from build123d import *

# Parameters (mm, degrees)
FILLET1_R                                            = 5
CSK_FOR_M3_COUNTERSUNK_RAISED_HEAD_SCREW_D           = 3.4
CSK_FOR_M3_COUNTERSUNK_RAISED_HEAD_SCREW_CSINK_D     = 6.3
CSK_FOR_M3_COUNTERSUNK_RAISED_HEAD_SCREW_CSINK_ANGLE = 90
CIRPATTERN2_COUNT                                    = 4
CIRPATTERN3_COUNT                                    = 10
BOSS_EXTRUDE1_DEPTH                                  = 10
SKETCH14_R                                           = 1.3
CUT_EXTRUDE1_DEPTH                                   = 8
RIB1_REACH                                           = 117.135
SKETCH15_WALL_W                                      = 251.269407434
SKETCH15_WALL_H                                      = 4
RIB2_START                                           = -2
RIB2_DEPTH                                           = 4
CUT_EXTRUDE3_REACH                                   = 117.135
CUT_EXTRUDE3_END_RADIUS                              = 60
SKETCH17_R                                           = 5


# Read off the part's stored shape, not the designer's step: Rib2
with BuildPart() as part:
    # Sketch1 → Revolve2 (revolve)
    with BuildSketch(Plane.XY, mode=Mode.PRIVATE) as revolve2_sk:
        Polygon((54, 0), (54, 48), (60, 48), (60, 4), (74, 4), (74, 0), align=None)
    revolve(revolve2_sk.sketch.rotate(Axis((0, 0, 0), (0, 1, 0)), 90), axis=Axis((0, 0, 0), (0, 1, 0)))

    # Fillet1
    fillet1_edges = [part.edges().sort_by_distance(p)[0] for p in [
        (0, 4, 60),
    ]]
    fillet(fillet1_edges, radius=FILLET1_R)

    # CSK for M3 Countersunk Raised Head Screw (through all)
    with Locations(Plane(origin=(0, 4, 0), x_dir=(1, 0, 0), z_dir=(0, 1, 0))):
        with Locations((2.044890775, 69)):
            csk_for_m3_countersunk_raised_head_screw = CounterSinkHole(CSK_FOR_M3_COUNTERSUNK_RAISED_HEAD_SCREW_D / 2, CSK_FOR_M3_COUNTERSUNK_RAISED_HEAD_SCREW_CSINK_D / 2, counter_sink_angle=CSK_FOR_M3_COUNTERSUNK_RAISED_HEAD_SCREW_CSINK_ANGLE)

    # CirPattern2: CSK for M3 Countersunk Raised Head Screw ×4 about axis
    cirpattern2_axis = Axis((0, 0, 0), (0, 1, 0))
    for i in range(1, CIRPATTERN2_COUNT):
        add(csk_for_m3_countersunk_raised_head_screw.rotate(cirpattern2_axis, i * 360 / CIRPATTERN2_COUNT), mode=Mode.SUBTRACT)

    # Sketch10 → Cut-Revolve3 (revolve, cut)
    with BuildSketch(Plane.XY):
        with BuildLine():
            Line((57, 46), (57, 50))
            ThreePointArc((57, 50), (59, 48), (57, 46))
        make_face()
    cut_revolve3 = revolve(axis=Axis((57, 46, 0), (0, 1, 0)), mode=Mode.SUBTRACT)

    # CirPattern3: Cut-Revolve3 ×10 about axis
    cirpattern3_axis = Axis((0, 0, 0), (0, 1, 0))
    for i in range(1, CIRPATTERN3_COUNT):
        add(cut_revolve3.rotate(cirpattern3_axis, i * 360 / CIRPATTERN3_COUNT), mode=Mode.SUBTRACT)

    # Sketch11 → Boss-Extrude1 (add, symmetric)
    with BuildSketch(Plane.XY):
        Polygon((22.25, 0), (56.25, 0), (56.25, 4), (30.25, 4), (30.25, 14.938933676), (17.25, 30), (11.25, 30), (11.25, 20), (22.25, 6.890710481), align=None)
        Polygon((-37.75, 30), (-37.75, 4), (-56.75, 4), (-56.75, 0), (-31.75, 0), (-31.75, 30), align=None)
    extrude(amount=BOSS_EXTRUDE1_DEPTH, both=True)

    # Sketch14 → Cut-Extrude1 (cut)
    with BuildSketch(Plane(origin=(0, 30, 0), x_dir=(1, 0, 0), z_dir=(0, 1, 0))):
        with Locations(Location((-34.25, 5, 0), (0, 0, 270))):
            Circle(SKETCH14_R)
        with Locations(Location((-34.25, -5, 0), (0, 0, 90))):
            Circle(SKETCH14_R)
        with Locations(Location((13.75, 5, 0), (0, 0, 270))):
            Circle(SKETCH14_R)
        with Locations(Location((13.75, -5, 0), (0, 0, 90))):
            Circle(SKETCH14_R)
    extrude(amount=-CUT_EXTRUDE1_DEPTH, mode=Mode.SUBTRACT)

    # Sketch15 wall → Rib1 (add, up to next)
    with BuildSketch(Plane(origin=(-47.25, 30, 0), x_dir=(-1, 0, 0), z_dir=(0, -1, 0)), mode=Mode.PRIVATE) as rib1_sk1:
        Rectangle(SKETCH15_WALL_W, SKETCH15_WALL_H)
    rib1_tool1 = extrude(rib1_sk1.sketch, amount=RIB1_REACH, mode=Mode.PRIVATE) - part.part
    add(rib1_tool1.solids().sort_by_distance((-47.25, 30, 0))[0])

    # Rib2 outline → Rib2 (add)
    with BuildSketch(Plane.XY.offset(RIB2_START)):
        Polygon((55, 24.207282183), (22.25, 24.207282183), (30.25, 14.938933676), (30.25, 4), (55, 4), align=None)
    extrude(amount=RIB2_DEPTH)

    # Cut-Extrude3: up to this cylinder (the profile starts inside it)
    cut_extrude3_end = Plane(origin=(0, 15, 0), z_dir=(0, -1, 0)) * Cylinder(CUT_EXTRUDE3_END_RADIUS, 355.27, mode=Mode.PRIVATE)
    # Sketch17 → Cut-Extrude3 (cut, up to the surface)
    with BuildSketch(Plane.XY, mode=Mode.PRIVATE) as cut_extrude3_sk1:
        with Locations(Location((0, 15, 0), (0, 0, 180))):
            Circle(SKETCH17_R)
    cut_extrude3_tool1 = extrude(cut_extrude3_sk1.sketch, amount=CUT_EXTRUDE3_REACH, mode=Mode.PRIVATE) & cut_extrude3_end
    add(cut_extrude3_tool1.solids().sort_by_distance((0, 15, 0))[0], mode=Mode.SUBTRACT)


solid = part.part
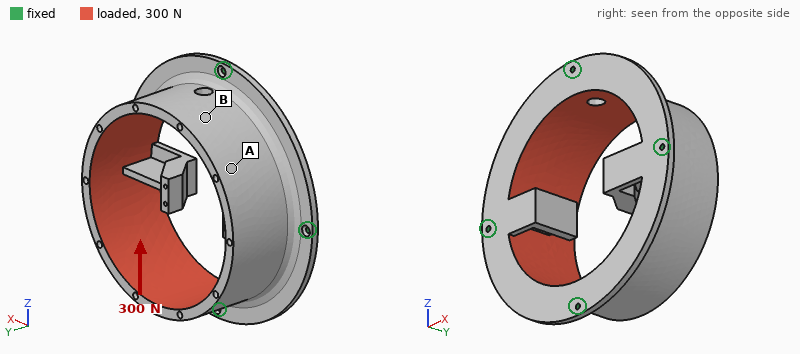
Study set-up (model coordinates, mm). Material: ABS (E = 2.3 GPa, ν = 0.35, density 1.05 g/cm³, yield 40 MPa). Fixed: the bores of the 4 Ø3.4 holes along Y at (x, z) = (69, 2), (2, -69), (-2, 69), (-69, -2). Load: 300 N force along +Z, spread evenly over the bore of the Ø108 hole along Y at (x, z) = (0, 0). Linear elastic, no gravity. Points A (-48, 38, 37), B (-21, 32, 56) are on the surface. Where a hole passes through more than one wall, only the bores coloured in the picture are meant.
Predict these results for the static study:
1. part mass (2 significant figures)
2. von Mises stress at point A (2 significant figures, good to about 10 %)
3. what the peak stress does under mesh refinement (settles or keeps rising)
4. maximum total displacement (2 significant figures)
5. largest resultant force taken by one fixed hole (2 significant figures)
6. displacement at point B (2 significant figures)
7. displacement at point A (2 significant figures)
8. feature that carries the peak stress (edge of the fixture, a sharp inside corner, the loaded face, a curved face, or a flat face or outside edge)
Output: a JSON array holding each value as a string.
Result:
["150 g", "0.37 MPa", "keeps rising", "69 µm", "92 N", "41 µm", "56 µm", "edge of the fixture"]
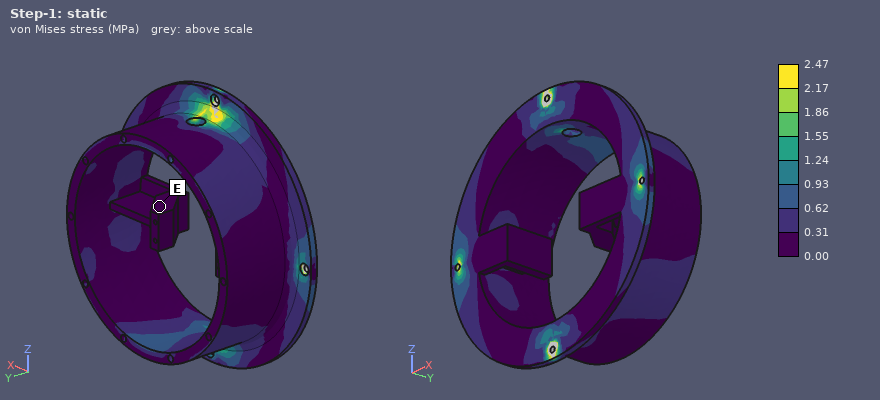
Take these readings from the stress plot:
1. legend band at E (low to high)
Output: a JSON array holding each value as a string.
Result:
["0.00 to 0.31 MPa"]
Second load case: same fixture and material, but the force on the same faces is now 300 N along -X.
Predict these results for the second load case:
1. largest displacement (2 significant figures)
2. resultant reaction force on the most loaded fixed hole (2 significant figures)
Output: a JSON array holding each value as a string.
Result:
["67 µm", "94 N"]
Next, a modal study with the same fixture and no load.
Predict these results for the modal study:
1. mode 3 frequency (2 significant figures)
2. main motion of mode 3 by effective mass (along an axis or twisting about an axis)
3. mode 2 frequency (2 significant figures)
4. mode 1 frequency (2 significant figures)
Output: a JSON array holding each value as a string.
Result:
["740 Hz", "along Y", "660 Hz", "490 Hz"]
